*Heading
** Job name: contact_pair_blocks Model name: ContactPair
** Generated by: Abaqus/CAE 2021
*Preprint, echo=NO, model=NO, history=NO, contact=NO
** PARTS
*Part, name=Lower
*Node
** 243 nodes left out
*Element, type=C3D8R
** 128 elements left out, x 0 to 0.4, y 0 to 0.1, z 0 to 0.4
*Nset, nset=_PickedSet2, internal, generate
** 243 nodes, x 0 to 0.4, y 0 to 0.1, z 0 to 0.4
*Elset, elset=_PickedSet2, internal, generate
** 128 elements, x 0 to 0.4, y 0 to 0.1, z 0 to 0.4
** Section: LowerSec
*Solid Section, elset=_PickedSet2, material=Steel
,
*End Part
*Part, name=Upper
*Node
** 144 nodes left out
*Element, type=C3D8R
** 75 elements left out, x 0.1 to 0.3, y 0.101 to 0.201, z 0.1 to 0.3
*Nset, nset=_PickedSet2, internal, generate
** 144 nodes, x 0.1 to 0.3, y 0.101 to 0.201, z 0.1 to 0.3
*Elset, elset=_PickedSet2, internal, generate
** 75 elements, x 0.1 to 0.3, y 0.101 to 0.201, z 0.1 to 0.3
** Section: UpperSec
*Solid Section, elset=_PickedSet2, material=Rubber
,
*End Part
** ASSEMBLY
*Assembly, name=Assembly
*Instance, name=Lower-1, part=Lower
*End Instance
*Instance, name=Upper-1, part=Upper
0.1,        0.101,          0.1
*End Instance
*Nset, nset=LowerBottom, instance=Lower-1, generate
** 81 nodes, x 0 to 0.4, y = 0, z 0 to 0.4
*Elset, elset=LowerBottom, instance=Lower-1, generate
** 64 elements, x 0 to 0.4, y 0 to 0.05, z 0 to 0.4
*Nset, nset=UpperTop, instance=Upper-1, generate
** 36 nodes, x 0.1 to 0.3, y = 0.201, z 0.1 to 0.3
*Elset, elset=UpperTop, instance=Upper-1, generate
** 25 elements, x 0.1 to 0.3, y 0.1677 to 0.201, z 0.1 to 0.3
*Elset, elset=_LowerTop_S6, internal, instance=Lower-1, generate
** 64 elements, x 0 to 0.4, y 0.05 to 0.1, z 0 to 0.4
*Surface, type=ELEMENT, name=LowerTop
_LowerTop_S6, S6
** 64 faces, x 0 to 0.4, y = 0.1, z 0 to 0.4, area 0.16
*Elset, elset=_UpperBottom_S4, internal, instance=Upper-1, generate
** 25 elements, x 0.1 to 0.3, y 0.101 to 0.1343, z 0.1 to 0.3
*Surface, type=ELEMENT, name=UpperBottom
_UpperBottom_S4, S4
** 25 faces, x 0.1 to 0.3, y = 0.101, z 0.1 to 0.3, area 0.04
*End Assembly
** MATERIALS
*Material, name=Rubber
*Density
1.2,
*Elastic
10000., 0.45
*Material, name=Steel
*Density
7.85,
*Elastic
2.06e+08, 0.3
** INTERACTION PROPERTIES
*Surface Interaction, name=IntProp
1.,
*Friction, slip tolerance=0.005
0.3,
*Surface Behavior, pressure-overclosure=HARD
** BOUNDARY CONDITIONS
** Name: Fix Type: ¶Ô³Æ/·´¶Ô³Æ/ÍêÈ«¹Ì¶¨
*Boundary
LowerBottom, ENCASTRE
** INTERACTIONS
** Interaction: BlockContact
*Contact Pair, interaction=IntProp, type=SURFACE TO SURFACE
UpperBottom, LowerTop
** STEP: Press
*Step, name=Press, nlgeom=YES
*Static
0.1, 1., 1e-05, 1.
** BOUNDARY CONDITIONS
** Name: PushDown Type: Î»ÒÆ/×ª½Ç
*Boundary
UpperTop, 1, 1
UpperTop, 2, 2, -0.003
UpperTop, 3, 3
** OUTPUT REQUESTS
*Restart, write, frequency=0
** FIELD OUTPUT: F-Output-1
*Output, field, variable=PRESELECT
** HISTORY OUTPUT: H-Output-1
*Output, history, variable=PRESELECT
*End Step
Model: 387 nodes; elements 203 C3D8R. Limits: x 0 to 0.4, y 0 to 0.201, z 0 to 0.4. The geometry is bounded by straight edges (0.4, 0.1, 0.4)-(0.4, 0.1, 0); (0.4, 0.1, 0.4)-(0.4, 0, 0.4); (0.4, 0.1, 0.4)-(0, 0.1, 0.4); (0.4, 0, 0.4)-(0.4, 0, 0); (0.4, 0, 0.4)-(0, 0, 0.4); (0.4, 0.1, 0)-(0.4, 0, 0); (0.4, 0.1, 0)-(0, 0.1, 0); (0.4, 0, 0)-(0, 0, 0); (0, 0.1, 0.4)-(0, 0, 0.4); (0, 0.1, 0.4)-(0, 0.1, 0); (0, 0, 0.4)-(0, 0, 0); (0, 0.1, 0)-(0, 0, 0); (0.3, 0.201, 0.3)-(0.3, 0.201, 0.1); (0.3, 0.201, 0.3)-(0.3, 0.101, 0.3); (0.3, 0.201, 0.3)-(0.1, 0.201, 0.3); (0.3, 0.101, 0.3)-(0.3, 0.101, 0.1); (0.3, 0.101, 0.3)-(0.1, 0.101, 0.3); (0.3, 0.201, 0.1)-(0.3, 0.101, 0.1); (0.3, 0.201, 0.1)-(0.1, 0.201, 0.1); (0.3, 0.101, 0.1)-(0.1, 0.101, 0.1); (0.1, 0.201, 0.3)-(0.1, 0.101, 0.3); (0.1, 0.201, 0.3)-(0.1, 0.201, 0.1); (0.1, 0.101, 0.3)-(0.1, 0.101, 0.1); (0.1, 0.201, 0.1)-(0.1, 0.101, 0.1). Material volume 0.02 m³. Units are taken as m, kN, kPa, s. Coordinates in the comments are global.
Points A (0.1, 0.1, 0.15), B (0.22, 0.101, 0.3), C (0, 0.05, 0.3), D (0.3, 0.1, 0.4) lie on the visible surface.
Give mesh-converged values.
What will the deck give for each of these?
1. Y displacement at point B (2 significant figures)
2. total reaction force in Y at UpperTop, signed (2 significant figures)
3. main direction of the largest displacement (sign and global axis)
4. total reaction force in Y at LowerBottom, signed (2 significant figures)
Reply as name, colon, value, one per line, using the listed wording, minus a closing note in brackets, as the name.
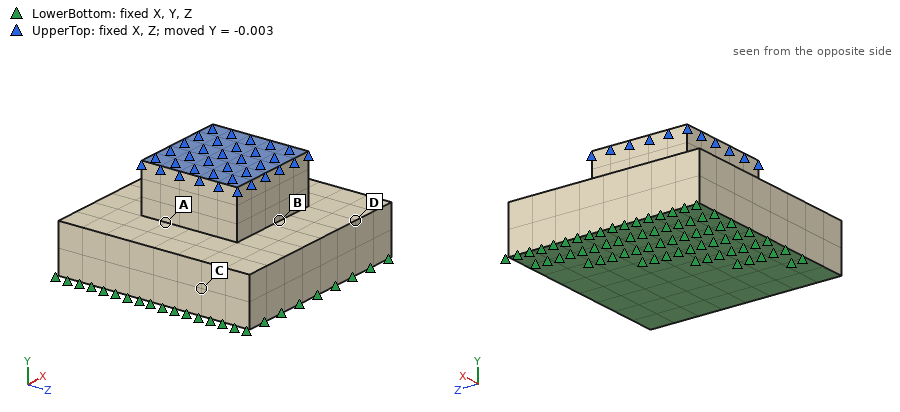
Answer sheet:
Y displacement at point B: -0.0010 m
total reaction force in Y at UpperTop, signed: -10 kN
main direction of the largest displacement: -Y
total reaction force in Y at LowerBottom, signed: 10 kN
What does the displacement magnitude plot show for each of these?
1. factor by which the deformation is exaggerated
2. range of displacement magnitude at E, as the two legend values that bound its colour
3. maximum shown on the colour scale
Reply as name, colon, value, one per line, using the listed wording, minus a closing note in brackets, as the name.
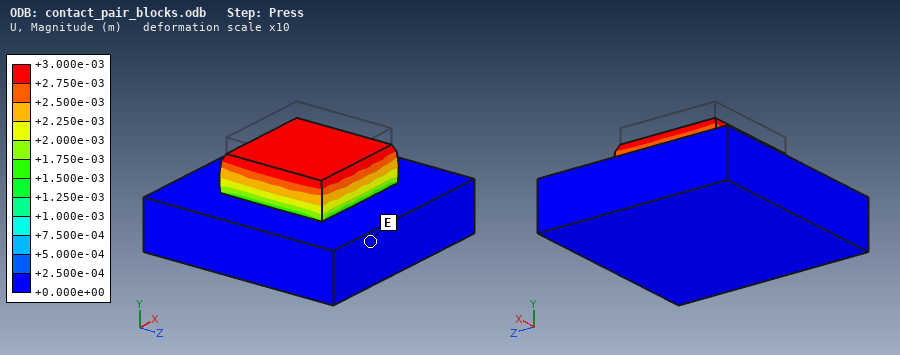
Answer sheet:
factor by which the deformation is exaggerated: 10
range of displacement magnitude at E, as the two legend values that bound its colour: +0.000e+00 to +2.500e-04 m
maximum shown on the colour scale: +3.000e-03 m
